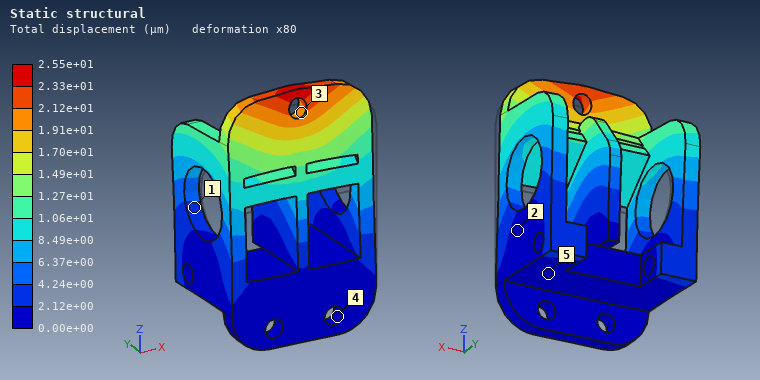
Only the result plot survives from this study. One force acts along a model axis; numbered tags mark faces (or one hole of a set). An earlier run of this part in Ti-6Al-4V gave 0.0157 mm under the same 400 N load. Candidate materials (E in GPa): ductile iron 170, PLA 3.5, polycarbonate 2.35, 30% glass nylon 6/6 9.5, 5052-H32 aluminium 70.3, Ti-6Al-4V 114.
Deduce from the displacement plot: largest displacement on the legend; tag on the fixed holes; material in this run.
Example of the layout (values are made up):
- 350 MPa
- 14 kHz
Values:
- 2.55e+01 µm
- 4
- 5052-H32 aluminium
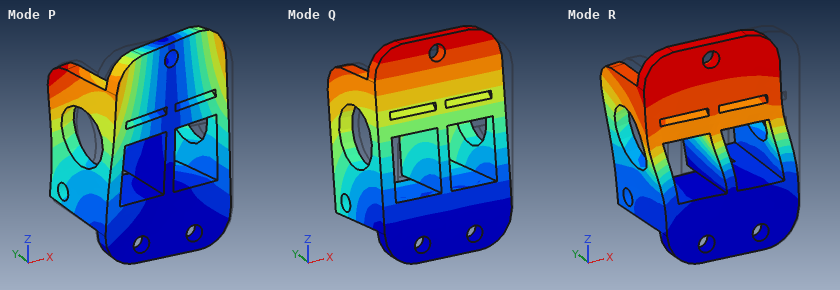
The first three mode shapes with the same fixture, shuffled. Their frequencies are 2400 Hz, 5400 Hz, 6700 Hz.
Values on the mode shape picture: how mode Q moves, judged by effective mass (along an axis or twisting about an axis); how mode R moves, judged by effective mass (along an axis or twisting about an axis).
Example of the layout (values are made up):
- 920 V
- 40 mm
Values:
- along Y
- along X
